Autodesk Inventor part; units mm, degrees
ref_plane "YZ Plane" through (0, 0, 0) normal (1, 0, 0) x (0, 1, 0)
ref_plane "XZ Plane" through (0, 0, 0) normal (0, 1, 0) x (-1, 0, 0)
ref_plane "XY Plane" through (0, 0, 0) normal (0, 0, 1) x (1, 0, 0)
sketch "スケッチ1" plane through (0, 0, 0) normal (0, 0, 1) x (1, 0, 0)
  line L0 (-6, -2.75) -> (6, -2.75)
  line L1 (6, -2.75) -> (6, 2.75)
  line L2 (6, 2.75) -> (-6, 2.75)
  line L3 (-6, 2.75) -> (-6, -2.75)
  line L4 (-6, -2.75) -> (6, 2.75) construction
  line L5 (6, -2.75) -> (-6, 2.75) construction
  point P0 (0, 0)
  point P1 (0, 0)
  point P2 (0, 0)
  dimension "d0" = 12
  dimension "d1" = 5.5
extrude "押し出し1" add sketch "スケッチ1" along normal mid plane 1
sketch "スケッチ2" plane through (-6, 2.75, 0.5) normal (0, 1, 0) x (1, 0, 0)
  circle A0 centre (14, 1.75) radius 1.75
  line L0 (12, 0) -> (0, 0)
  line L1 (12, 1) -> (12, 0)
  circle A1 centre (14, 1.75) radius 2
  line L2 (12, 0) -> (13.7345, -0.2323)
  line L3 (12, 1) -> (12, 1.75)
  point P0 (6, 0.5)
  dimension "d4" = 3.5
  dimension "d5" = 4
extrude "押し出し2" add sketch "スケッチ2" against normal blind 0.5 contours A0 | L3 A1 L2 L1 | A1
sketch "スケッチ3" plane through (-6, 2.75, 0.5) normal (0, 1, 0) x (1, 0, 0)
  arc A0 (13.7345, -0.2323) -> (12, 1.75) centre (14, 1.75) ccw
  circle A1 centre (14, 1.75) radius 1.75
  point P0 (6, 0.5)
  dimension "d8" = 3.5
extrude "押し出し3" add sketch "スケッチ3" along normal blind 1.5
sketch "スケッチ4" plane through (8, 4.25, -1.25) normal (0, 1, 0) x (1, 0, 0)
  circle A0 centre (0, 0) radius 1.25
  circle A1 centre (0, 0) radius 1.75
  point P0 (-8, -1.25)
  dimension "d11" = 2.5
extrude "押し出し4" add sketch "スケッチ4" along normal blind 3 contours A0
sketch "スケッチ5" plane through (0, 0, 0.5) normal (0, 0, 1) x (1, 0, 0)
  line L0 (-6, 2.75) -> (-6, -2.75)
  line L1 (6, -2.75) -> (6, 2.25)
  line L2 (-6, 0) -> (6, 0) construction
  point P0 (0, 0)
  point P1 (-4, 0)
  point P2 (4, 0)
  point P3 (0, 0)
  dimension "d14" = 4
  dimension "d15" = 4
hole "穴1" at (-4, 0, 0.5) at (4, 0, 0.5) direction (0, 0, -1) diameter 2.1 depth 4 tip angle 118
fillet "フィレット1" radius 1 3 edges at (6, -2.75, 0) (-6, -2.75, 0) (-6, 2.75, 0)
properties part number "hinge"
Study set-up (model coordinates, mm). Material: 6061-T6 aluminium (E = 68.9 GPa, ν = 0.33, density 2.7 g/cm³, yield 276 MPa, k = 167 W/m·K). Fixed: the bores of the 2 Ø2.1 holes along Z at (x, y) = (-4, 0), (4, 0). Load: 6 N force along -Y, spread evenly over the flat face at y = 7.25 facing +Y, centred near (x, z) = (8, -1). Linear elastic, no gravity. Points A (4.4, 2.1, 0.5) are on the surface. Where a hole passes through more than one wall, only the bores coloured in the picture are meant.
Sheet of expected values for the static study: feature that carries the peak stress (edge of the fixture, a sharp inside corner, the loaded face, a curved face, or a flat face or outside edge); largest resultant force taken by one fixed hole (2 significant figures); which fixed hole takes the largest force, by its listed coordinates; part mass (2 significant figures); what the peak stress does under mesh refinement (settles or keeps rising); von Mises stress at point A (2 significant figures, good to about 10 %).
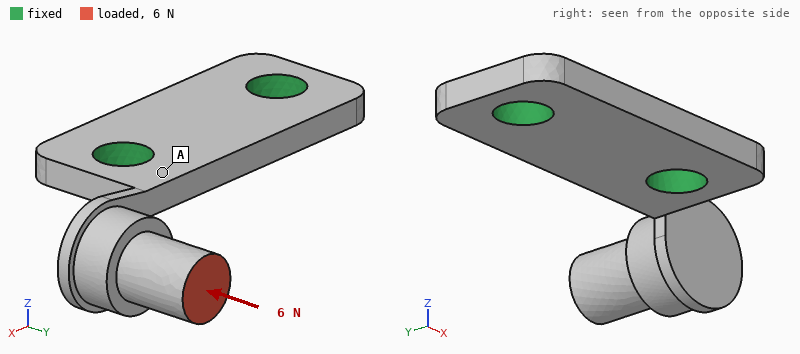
a sharp inside corner
7.3 N
(4, 0)
0.25 g
keeps rising
22 MPa
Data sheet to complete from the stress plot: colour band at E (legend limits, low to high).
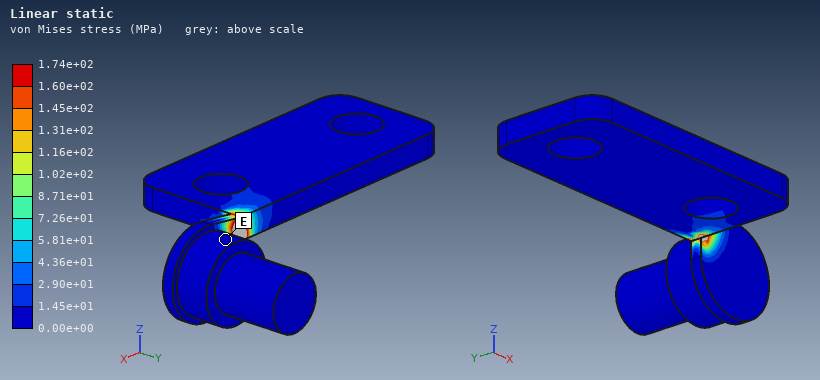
0.00e+00 to 1.45e+01 MPa
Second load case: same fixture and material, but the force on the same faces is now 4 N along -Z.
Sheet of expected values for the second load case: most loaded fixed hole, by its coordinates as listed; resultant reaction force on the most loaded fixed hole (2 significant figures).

(4, 0)
4.5 N
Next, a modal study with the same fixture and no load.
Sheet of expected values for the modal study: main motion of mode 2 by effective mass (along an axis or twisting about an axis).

along Z
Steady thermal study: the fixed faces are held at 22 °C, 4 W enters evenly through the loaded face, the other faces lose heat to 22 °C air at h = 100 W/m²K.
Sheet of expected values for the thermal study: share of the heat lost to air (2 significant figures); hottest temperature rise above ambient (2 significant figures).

12 %
84 K
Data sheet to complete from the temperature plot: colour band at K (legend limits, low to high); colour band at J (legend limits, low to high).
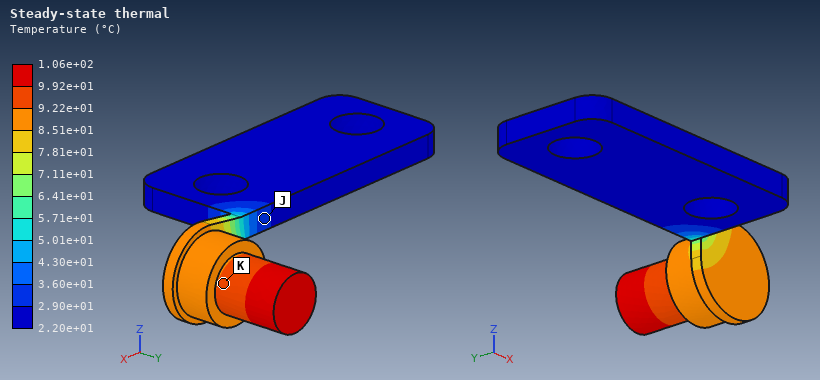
9.22e+01 to 9.92e+01 °C
2.90e+01 to 3.60e+01 °C
